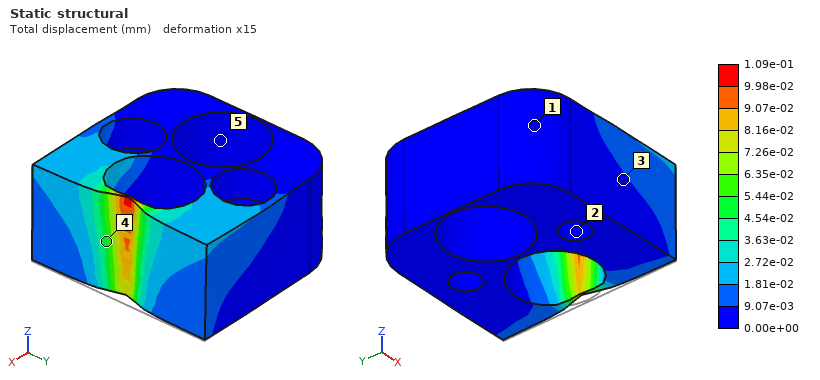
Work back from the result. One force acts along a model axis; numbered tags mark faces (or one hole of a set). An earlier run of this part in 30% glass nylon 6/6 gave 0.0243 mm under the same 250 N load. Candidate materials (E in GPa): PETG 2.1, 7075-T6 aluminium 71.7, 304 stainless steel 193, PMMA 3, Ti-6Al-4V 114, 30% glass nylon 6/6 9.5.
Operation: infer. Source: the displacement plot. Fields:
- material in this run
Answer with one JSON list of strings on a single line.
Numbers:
["PETG"]
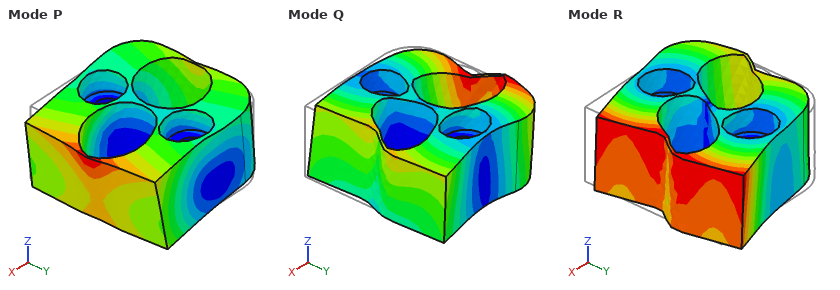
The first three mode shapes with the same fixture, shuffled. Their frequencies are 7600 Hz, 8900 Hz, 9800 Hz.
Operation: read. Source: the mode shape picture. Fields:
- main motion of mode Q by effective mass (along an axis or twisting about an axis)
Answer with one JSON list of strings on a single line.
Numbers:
["along Y"]
